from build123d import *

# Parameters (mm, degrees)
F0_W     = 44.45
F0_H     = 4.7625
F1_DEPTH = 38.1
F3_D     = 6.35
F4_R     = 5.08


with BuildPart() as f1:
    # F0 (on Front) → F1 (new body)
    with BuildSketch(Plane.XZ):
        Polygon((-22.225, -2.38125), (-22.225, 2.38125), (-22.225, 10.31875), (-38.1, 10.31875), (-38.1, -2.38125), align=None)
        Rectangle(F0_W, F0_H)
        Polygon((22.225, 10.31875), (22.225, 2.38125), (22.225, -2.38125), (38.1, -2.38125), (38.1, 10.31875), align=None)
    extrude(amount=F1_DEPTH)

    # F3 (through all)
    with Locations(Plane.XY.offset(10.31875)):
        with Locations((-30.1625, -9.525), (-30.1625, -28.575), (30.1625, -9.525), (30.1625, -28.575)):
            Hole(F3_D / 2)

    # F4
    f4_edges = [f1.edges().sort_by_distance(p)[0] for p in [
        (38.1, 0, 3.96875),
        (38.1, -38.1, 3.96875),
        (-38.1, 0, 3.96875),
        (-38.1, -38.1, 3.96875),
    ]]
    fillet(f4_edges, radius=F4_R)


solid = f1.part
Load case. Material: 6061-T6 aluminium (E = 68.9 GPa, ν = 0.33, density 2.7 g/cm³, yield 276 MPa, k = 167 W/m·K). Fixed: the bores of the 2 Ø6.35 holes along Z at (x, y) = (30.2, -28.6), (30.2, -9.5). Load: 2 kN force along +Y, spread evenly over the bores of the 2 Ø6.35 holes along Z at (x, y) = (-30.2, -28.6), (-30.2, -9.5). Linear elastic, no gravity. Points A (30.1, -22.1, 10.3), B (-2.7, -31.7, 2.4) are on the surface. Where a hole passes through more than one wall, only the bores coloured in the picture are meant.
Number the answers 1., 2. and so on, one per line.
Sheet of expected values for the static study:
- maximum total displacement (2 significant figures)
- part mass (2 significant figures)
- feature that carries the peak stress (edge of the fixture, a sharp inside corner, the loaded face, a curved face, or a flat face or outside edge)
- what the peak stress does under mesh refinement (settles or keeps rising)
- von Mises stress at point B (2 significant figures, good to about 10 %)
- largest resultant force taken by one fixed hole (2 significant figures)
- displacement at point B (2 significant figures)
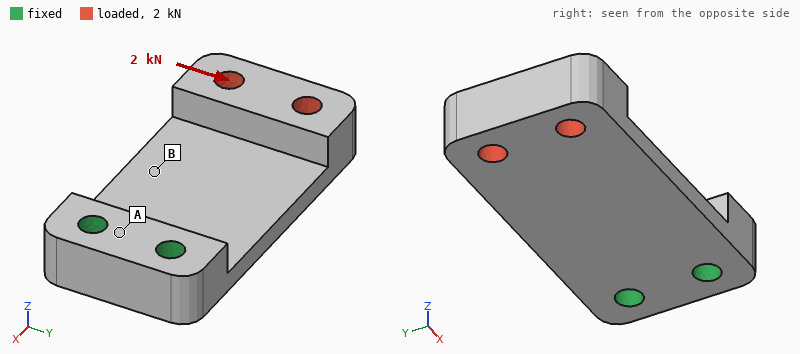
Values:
1. 0.28 mm
2. 58 g
3. edge of the fixture
4. keeps rising
5. 70 MPa
6. 5.0 kN
7. 0.091 mm
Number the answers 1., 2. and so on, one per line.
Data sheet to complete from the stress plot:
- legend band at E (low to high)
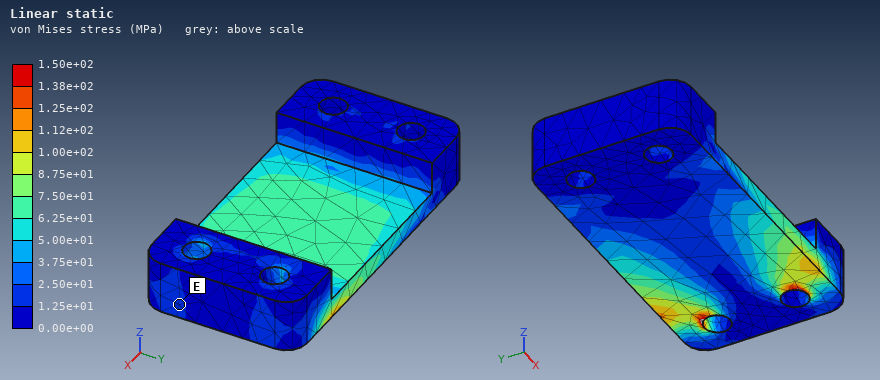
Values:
1. 1.25e+01 to 2.50e+01 MPa
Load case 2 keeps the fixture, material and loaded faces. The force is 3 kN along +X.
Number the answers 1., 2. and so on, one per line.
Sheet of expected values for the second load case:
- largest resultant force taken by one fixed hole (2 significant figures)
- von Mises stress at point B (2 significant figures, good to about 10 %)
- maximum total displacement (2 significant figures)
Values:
1. 1.5 kN
2. 97 MPa
3. 0.92 mm
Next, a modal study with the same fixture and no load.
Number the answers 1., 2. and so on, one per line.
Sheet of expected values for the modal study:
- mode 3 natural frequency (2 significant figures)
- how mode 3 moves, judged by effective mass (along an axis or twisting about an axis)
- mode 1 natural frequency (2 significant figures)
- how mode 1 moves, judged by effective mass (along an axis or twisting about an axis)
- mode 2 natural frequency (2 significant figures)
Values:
1. 4400 Hz
2. along Y
3. 720 Hz
4. along Z
5. 2600 Hz
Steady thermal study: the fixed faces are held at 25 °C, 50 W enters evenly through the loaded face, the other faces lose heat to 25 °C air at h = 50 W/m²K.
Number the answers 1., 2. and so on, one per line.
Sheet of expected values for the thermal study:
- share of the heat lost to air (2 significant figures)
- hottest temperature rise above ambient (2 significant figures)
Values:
1. 28 %
2. 71 K
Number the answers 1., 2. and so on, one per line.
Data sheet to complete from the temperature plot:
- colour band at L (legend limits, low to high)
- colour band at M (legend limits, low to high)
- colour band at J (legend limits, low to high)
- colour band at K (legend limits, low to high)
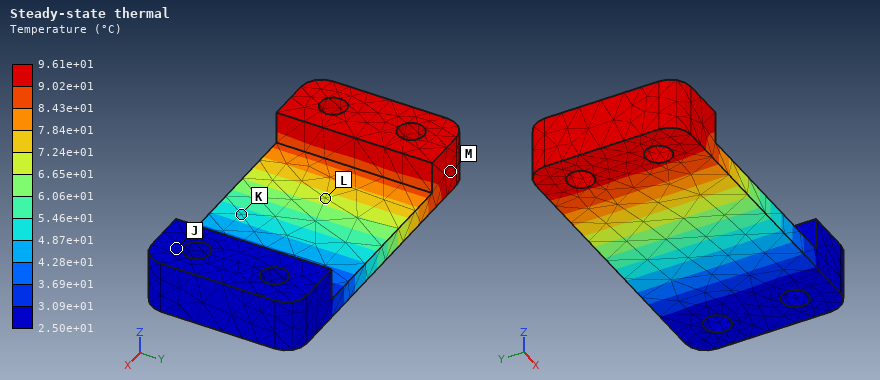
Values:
1. 6.65e+01 to 7.24e+01 °C
2. 9.02e+01 to 9.61e+01 °C
3. 2.50e+01 to 3.09e+01 °C
4. 4.87e+01 to 5.46e+01 °C
